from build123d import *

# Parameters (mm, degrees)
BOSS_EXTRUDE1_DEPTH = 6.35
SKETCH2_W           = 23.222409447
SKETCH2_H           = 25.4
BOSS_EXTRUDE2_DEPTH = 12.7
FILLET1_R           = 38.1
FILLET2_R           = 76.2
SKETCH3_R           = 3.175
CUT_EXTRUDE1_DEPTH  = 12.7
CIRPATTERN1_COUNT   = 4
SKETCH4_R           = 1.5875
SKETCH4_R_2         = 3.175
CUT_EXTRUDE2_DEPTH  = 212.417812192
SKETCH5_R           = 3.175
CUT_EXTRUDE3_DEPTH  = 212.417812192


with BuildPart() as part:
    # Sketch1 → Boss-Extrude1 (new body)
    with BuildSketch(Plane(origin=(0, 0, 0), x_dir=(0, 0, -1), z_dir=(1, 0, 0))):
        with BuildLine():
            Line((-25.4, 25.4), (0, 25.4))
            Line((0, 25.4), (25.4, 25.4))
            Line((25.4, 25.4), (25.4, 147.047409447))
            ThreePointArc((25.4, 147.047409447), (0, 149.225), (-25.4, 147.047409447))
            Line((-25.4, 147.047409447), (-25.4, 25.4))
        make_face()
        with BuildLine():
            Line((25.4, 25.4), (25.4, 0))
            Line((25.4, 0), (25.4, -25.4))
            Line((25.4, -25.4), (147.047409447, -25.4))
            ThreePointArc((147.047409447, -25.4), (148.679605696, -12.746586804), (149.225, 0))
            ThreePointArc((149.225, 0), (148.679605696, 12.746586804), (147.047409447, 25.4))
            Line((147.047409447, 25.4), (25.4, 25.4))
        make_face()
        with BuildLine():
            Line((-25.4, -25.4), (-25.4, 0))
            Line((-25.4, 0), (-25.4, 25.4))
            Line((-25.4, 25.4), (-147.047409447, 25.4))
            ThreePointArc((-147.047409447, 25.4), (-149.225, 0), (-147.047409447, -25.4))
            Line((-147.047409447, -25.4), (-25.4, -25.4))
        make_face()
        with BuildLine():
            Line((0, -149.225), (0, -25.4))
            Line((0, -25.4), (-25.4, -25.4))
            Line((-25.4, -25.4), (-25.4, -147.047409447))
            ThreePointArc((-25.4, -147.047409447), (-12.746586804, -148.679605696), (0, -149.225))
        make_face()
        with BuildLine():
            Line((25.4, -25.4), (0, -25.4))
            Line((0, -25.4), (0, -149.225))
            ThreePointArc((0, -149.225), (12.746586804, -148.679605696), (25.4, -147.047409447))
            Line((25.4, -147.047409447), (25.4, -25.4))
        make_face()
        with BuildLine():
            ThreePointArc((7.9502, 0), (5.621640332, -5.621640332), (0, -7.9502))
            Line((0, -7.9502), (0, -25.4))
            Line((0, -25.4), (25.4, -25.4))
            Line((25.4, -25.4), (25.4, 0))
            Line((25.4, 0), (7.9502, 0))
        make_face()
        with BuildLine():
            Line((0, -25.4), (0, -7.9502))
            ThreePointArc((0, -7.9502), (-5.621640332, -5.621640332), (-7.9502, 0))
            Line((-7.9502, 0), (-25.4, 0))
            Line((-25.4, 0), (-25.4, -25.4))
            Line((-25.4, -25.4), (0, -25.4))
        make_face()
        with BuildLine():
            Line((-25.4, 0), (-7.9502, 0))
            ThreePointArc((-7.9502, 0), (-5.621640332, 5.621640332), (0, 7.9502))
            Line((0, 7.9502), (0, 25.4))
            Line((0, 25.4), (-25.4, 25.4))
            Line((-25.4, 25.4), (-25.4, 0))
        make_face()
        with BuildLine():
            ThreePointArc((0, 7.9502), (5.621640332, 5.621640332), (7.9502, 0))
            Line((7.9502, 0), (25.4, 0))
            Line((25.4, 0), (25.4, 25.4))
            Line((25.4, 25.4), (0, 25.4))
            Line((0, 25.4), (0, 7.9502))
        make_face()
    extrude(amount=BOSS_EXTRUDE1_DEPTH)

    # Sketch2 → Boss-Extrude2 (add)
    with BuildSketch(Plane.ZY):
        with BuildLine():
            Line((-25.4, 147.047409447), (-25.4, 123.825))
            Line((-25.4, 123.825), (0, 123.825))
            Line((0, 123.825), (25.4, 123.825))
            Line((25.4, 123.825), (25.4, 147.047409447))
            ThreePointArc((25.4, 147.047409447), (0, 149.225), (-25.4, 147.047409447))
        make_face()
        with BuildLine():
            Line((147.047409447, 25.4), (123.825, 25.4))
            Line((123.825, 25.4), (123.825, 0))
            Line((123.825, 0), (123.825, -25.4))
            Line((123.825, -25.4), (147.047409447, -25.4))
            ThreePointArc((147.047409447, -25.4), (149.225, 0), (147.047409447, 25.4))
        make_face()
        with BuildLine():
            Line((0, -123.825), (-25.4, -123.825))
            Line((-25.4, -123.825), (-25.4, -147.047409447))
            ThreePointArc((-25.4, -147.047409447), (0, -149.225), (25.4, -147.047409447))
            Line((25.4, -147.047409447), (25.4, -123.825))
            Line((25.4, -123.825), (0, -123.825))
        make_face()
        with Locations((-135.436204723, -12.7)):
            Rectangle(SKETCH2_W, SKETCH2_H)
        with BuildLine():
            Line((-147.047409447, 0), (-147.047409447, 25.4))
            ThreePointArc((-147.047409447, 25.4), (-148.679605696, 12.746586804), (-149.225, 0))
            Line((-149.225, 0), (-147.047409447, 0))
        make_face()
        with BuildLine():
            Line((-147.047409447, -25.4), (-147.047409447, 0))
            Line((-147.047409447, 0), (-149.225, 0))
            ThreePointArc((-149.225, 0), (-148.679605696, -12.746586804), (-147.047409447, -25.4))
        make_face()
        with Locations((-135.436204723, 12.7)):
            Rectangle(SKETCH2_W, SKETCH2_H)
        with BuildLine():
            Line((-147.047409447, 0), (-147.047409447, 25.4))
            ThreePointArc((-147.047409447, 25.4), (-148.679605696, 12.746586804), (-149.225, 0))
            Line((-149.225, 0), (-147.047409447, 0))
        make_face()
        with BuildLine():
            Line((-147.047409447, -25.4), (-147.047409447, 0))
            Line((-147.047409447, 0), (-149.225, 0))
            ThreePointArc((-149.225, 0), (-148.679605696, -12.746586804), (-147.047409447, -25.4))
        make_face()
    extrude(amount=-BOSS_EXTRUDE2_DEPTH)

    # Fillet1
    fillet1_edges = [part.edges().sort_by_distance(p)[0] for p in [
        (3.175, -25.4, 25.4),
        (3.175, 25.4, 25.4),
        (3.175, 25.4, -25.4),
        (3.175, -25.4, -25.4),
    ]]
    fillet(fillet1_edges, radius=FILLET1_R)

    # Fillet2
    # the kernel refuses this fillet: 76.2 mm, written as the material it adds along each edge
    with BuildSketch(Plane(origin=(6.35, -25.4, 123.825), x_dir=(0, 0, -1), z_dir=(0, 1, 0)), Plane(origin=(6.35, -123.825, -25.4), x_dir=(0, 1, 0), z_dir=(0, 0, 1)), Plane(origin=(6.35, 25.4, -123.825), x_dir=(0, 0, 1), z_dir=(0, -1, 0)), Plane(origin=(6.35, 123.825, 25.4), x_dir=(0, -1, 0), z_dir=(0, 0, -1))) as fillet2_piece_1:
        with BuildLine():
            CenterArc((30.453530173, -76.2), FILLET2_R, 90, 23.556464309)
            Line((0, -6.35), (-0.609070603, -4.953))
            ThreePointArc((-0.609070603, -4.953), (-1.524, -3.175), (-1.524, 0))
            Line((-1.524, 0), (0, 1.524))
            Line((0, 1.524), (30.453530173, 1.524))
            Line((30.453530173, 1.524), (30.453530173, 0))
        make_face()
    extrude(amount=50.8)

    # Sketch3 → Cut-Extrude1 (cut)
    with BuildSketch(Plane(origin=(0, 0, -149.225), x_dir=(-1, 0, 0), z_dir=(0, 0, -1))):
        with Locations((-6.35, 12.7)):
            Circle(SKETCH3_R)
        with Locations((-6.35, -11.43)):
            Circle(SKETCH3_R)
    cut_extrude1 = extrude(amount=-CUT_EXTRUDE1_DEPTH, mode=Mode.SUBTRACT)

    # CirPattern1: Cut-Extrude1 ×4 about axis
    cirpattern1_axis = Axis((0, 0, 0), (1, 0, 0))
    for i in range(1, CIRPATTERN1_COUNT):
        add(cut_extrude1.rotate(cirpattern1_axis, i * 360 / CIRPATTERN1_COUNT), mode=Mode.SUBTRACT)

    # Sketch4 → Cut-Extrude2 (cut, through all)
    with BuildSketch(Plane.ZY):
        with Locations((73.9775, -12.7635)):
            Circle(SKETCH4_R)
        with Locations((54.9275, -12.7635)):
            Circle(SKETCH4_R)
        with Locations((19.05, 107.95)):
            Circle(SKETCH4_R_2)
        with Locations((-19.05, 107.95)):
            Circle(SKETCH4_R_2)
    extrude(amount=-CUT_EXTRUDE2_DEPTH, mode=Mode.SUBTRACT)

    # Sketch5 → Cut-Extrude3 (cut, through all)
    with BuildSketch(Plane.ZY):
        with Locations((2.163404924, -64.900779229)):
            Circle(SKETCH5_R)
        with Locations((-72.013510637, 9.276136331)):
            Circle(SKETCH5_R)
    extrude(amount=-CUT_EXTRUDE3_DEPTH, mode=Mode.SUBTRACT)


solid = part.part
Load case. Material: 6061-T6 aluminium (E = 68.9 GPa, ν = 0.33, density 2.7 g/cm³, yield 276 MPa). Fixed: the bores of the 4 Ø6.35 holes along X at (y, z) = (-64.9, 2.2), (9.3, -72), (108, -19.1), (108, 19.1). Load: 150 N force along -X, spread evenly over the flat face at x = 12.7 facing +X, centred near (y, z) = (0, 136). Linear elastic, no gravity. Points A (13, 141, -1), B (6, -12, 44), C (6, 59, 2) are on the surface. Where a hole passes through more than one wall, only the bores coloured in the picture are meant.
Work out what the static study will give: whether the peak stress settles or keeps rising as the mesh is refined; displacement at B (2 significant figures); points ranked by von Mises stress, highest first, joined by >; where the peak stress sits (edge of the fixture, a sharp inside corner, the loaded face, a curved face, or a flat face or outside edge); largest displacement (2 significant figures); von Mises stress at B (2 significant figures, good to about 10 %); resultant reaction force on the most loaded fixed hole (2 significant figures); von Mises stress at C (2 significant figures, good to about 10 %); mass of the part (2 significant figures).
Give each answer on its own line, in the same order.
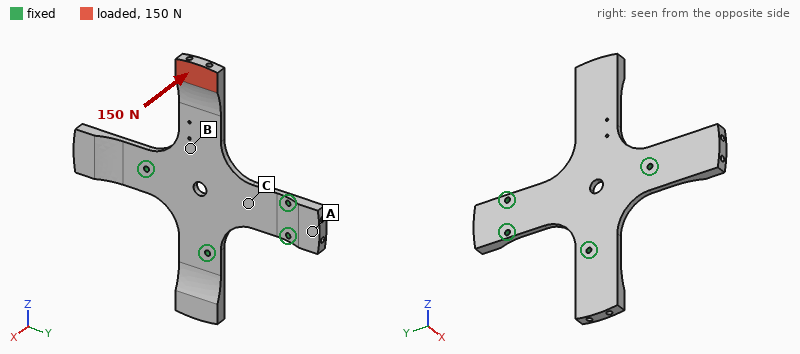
keeps rising
0.26 mm
B > C > A
edge of the fixture
1.7 mm
35 MPa
180 N
14 MPa
600 g
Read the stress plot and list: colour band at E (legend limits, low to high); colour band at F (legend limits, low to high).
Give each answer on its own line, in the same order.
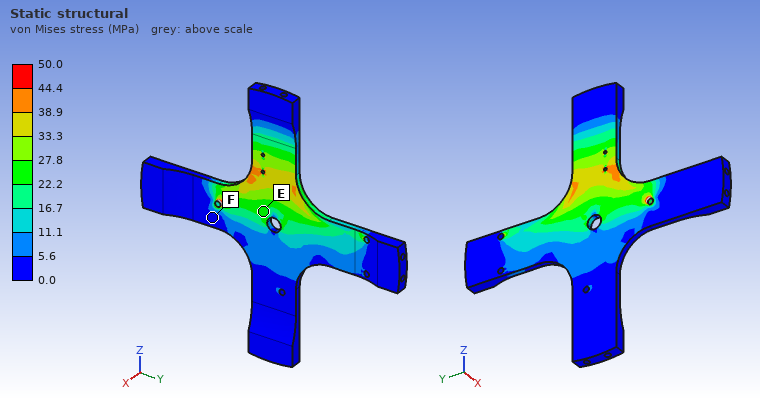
22.2 to 27.8 MPa
0.0 to 5.6 MPa
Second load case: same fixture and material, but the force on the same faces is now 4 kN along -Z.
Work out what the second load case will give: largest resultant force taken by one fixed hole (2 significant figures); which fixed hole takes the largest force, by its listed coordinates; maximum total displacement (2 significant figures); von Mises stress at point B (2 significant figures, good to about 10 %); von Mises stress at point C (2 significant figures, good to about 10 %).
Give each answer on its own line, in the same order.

2.2 kN
(9.3, -72)
4.6 mm
100 MPa
29 MPa
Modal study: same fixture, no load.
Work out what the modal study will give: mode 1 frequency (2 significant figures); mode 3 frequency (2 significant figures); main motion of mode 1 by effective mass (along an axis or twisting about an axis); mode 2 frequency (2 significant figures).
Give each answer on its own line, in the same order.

190 Hz
640 Hz
along X
550 Hz
